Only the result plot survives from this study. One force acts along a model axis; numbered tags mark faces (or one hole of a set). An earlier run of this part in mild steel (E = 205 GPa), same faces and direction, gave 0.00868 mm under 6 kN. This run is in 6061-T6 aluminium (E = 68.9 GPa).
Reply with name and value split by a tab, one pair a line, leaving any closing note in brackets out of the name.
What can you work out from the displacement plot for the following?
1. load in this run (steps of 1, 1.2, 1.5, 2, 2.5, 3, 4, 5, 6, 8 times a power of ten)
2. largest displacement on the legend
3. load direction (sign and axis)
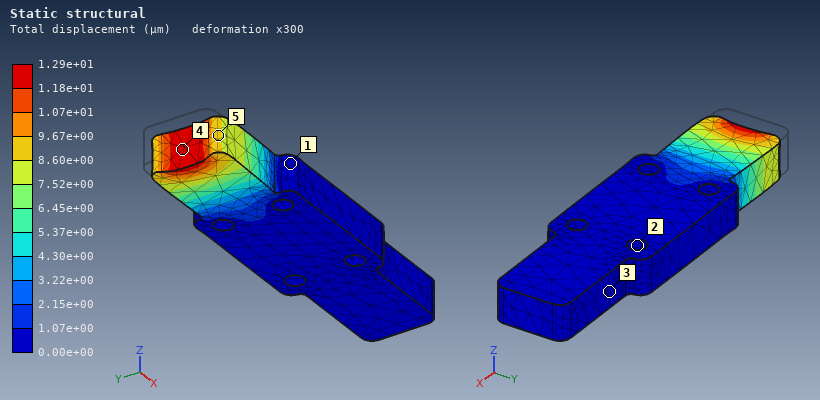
load in this run	3 kN
largest displacement on the legend	1.29e+01 µm
load direction	+X
